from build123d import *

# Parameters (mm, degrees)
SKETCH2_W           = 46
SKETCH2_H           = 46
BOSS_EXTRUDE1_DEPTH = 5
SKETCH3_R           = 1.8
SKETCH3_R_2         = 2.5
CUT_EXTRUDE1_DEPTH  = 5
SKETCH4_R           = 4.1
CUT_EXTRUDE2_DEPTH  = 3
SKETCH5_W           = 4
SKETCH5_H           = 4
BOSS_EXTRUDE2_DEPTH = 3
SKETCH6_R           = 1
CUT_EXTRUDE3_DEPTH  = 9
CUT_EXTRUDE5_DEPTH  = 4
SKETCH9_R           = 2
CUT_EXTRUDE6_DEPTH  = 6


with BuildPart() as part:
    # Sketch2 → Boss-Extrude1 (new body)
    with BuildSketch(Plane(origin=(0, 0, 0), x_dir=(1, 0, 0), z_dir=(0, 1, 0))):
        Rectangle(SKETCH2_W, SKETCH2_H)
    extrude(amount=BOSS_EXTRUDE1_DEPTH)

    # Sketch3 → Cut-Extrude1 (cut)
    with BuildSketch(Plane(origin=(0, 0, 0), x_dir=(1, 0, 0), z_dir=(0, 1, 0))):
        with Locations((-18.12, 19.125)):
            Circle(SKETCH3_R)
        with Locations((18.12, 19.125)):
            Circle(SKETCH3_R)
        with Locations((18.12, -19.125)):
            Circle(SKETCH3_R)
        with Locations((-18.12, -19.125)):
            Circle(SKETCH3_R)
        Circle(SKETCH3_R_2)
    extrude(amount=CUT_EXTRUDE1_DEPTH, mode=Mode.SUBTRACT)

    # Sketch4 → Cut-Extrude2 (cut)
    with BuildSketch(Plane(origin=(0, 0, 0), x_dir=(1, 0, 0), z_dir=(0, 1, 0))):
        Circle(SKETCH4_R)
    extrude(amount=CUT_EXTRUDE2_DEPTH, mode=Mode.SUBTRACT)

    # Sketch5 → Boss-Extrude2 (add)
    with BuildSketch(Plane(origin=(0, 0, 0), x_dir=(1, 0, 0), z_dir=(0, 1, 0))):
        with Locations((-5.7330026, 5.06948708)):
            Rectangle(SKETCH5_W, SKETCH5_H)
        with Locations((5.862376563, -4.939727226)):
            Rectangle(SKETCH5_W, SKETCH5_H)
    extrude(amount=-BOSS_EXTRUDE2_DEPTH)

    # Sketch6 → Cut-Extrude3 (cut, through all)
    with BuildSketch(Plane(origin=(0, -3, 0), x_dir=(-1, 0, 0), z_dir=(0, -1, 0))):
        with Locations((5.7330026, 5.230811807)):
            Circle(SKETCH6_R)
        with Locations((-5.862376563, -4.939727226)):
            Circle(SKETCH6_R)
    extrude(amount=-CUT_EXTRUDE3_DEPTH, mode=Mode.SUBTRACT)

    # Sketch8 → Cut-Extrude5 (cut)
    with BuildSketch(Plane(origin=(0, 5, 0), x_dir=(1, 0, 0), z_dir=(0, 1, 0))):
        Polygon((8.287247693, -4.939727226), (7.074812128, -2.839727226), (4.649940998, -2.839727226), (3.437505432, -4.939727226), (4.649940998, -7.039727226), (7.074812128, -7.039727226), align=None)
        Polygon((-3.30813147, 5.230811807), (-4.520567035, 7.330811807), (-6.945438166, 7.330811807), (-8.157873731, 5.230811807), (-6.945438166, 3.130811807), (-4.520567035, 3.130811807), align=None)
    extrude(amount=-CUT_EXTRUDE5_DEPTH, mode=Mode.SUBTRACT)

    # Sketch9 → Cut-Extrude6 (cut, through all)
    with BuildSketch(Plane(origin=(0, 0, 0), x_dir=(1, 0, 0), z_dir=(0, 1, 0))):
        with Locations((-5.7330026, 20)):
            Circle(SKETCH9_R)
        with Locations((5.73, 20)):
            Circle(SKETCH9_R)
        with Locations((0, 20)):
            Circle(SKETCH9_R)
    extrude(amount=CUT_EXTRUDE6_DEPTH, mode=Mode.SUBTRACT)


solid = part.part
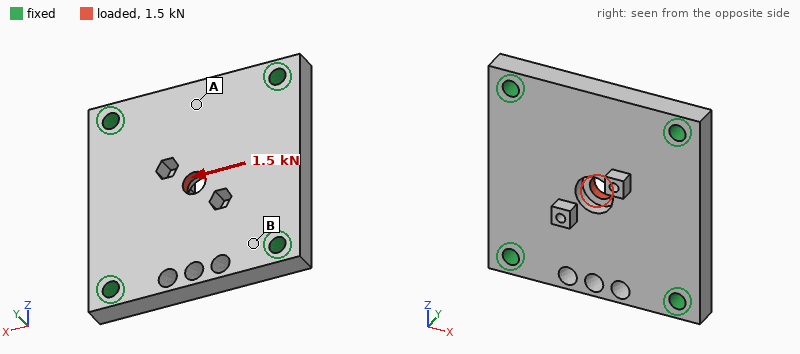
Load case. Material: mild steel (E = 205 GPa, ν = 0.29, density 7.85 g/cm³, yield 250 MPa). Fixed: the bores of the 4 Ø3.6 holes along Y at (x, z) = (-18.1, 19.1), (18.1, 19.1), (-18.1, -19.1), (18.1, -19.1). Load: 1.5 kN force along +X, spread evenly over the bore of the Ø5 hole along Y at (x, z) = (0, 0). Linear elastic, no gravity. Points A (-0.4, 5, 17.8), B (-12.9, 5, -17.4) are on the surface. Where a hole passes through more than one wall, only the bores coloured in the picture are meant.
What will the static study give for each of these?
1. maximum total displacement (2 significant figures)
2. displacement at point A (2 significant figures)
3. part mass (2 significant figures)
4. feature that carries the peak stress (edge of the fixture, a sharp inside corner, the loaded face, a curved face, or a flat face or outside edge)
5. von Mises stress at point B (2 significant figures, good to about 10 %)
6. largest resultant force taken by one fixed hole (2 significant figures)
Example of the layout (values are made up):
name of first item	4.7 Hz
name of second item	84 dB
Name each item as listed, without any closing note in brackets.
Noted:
maximum total displacement	2.3 µm
displacement at point A	0.35 µm
part mass	78 g
feature that carries the peak stress	the loaded face
von Mises stress at point B	9.1 MPa
largest resultant force taken by one fixed hole	430 N
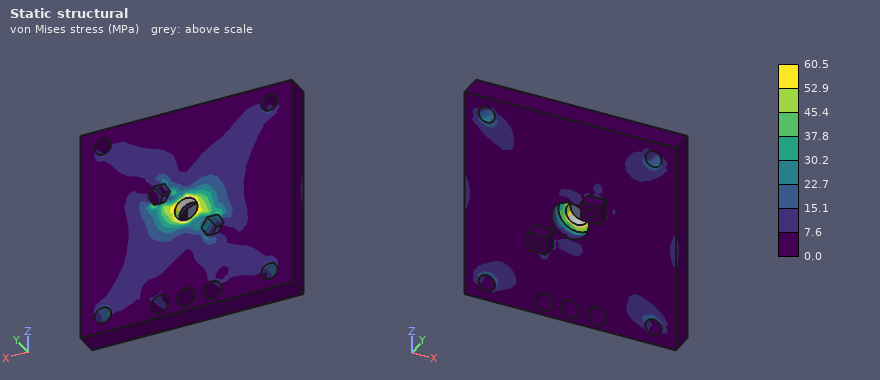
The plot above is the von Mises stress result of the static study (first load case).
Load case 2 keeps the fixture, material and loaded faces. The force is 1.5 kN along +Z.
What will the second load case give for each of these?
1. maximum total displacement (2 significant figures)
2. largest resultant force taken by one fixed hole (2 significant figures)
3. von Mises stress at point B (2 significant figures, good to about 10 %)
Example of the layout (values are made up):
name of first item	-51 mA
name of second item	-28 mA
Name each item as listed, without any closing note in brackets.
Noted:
maximum total displacement	2.2 µm
largest resultant force taken by one fixed hole	430 N
von Mises stress at point B	6.7 MPa
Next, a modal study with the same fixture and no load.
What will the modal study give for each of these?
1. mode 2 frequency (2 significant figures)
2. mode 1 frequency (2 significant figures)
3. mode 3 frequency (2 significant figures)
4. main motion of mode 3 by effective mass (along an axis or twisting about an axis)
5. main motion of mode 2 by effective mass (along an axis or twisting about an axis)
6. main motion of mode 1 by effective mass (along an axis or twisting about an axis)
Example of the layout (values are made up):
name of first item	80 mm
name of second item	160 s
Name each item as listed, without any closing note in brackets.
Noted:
mode 2 frequency	18 kHz
mode 1 frequency	12 kHz
mode 3 frequency	20 kHz
main motion of mode 3 by effective mass	twisting about X
main motion of mode 2 by effective mass	twisting about Z
main motion of mode 1 by effective mass	along Y
